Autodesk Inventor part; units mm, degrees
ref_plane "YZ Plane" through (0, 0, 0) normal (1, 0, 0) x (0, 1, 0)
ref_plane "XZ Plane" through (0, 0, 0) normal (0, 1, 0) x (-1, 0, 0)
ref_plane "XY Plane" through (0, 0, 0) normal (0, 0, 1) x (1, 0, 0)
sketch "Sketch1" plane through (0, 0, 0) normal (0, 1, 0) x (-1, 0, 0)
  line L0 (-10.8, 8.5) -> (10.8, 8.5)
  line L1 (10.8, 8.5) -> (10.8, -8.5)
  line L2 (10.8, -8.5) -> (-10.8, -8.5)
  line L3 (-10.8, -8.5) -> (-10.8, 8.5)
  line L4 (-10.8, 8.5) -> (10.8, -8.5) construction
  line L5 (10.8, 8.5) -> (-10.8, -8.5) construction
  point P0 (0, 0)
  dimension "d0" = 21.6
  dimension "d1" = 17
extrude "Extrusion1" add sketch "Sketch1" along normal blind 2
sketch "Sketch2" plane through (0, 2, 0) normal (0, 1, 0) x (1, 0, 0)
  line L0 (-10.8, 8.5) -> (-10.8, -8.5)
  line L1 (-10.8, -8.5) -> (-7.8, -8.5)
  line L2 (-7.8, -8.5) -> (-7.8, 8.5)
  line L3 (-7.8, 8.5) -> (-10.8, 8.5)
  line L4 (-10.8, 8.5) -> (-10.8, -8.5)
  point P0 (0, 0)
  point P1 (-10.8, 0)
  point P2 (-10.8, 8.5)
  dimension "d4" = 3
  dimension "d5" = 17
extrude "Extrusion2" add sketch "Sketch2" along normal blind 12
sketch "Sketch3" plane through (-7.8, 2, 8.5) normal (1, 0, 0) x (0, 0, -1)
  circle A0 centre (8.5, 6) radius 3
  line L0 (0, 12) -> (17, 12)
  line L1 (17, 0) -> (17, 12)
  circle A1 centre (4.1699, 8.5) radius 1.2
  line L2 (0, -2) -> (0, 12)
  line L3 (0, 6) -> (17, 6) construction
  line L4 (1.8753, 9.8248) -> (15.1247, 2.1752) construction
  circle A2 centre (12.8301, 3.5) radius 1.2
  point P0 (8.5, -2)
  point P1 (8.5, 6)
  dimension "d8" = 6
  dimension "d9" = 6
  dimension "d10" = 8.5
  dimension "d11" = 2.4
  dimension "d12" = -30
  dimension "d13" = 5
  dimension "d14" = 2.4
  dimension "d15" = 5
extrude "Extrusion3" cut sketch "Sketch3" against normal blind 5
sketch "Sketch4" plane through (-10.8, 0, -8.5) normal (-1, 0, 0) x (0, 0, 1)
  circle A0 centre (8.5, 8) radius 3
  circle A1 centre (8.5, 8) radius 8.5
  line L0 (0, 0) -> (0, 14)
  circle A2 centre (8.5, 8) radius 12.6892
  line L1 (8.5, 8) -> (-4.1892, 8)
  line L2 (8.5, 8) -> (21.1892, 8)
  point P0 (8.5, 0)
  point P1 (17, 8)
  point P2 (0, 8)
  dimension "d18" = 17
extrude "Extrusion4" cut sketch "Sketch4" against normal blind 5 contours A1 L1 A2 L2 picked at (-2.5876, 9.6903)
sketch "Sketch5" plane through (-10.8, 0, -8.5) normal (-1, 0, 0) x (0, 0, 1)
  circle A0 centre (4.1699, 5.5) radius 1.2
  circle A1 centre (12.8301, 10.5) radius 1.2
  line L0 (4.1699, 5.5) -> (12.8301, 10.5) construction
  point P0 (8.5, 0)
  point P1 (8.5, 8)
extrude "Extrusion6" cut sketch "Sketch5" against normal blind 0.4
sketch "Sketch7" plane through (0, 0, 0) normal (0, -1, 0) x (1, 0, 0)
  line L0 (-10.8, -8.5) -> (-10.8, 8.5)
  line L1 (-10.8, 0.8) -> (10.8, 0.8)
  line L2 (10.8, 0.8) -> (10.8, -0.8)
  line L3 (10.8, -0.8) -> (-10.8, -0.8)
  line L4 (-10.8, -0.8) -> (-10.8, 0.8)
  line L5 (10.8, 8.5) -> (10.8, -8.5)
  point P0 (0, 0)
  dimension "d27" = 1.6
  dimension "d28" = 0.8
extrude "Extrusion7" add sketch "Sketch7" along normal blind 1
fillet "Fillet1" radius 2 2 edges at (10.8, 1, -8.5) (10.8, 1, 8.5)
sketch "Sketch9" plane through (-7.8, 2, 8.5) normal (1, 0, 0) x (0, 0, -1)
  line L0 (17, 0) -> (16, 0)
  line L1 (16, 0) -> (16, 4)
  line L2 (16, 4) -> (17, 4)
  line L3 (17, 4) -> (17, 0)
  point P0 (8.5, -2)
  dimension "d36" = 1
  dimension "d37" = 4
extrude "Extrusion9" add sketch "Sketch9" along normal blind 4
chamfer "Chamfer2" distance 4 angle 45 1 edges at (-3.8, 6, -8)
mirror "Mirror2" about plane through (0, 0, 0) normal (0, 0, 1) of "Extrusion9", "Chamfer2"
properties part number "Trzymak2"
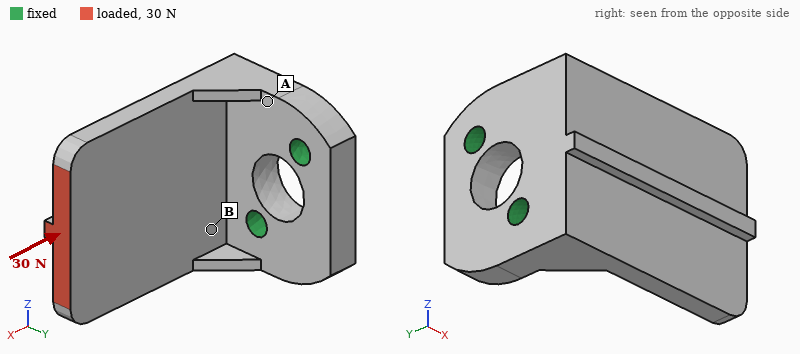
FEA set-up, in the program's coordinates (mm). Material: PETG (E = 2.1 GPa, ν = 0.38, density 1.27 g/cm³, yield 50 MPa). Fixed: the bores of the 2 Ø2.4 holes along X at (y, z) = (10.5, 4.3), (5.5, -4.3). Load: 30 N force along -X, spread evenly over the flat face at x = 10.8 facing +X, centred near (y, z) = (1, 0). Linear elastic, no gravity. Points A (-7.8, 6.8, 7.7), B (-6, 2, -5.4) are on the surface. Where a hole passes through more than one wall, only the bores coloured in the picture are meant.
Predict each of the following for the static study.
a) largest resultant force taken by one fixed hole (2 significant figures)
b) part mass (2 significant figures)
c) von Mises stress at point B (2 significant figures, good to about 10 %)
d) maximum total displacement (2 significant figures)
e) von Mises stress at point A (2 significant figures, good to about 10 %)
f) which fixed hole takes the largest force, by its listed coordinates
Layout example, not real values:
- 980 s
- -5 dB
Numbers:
- 23 N
- 1.6 g
- 1.7 MPa
- 0.20 mm
- 4.0 MPa
- (5.5, -4.3)
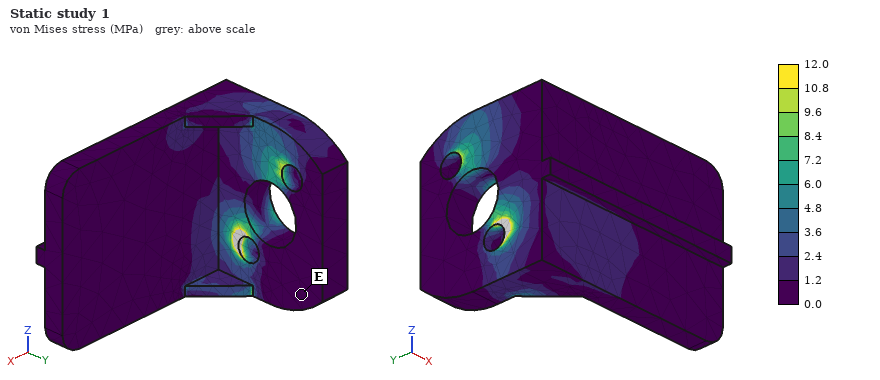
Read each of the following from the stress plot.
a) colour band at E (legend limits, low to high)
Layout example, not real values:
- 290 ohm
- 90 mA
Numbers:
- 0.0 to 1.2 MPa
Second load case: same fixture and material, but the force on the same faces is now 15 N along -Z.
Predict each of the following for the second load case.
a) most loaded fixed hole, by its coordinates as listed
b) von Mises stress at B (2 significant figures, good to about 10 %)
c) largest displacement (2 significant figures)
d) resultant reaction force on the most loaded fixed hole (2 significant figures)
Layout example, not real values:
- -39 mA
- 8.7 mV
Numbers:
- (5.5, -4.3)
- 5.2 MPa
- 0.29 mm
- 22 N
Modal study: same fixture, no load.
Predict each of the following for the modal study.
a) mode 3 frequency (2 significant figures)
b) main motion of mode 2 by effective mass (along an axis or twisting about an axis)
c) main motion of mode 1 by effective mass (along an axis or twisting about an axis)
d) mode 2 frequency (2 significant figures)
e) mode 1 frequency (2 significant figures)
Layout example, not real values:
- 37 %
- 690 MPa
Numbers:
- 3300 Hz
- along Z
- along Y
- 2100 Hz
- 1100 Hz
